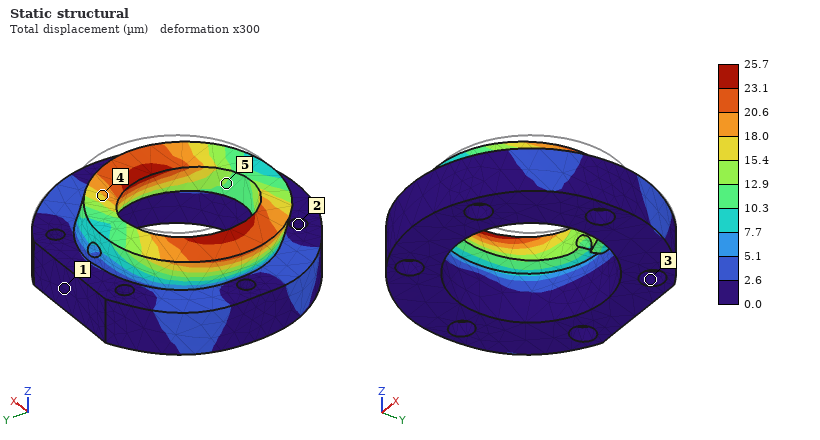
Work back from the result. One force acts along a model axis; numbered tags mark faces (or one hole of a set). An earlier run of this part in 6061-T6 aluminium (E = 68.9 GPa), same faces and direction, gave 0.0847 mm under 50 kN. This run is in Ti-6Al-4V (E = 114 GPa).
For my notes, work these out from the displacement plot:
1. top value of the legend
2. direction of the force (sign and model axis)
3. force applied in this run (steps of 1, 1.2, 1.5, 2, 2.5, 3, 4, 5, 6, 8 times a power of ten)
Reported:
25.7 µm
-X
25 kN
